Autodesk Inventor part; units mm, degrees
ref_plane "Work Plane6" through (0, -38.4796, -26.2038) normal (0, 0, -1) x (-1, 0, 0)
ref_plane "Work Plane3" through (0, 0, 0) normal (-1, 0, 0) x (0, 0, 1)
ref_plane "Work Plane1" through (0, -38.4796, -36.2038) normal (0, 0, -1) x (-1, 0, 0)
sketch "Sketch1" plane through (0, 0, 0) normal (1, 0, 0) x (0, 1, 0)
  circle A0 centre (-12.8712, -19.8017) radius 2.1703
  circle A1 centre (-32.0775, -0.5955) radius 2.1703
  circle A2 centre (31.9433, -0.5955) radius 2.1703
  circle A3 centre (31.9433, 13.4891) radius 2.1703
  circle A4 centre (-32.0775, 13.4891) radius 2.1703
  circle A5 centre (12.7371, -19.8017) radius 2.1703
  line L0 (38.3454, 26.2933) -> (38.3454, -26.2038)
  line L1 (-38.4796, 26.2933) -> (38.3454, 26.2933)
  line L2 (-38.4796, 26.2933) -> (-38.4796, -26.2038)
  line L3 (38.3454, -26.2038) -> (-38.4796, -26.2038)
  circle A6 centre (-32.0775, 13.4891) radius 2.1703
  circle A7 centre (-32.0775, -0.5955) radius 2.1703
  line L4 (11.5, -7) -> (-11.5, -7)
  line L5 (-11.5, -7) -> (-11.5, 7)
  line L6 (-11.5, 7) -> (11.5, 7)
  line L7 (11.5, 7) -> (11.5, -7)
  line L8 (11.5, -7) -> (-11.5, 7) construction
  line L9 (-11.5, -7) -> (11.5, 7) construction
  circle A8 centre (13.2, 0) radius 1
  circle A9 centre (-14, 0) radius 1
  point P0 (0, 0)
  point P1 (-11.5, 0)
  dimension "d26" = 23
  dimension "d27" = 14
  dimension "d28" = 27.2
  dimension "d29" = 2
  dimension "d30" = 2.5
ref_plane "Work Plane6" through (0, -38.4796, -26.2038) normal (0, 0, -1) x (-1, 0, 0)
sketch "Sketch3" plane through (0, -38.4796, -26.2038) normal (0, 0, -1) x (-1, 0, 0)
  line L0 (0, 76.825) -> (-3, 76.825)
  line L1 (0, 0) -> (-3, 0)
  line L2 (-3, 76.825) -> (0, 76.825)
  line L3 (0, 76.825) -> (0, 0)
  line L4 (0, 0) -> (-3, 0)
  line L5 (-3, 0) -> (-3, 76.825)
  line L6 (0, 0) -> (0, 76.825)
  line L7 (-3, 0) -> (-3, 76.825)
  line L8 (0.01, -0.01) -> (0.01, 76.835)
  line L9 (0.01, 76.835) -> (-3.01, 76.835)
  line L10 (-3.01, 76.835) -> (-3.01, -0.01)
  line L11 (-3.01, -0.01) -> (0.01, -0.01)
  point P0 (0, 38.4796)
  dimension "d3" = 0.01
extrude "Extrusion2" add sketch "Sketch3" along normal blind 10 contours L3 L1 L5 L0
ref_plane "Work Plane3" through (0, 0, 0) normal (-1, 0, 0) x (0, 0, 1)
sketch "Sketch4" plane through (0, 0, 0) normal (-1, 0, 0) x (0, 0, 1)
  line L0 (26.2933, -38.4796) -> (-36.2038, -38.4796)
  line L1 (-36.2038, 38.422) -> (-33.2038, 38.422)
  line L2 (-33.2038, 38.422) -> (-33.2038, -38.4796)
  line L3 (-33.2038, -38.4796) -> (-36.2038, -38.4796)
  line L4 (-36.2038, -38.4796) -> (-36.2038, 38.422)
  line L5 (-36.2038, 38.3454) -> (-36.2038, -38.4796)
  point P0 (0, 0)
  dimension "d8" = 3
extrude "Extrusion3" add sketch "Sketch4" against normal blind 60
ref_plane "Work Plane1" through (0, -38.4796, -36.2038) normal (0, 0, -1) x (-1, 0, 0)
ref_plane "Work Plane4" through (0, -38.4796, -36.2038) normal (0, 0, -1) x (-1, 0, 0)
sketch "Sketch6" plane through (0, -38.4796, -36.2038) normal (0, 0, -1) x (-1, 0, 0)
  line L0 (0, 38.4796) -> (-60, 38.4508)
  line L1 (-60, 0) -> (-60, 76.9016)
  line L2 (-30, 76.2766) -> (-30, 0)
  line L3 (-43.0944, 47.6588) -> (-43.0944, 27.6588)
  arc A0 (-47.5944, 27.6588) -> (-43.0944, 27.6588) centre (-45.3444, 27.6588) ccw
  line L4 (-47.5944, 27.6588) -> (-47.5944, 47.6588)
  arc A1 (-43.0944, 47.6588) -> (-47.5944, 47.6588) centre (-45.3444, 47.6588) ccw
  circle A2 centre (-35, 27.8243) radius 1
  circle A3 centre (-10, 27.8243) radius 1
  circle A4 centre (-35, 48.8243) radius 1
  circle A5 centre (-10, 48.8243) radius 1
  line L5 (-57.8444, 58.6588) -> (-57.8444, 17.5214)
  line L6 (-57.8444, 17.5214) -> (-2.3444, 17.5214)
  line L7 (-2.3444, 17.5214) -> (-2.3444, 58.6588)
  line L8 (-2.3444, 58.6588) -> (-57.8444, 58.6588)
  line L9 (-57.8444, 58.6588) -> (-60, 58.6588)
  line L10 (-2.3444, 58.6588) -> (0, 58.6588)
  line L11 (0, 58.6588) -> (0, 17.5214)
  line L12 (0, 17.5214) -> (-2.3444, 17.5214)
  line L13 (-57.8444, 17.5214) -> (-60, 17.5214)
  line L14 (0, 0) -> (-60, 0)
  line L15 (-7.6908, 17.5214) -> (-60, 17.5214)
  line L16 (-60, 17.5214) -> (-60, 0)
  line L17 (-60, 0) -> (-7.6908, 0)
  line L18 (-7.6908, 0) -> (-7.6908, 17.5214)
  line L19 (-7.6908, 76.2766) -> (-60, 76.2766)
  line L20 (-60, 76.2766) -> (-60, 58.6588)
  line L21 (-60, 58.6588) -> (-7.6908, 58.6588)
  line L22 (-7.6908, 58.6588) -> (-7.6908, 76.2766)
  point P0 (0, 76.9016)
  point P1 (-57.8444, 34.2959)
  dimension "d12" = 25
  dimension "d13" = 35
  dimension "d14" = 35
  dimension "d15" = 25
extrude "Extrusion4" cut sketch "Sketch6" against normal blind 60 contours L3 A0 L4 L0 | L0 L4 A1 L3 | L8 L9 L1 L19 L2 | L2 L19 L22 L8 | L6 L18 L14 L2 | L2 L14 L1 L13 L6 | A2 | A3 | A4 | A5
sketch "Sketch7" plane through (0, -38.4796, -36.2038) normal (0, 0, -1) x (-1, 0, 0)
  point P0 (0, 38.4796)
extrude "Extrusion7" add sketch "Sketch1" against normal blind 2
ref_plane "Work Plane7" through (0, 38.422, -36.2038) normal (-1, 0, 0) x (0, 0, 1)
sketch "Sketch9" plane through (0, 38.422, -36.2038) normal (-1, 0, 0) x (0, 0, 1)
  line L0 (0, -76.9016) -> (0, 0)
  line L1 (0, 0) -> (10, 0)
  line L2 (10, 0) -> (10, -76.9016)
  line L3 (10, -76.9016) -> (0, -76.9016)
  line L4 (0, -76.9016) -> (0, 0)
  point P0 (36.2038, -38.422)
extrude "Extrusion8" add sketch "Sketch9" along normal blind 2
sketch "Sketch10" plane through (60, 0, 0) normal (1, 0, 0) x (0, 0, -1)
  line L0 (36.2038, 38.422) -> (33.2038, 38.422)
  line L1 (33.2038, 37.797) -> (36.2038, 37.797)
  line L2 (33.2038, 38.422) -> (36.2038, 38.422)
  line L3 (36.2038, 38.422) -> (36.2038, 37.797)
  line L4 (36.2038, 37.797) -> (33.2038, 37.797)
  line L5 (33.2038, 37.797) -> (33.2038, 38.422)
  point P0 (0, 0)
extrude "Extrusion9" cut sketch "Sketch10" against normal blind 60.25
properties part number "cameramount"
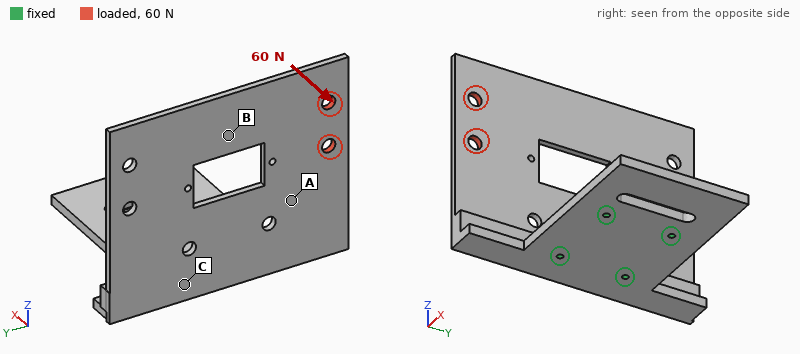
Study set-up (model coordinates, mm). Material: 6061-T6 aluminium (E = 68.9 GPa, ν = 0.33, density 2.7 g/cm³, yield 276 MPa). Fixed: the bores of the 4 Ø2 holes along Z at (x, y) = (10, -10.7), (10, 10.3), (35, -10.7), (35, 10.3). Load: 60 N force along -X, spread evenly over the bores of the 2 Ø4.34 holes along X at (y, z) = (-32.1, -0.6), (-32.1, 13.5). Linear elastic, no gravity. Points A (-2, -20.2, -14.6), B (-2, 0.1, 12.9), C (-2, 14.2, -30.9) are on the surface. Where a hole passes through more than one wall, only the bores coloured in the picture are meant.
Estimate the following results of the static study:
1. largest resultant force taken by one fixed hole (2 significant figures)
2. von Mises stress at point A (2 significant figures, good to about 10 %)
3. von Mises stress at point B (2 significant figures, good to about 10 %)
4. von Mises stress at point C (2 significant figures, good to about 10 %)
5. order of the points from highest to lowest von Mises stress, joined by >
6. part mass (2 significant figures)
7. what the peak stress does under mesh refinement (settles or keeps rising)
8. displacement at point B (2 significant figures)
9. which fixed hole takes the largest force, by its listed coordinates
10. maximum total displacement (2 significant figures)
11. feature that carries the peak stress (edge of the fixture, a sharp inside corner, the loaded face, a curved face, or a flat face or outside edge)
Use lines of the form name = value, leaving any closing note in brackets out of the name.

largest resultant force taken by one fixed hole = 72 N
von Mises stress at point A = 42 MPa
von Mises stress at point B = 17 MPa
von Mises stress at point C = 8.4 MPa
order of the points from highest to lowest von Mises stress, joined by > = A > B > C
part mass = 49 g
what the peak stress does under mesh refinement = keeps rising
displacement at point B = 0.46 mm
which fixed hole takes the largest force, by its listed coordinates = (10, -10.7)
maximum total displacement = 1.1 mm
feature that carries the peak stress = edge of the fixture
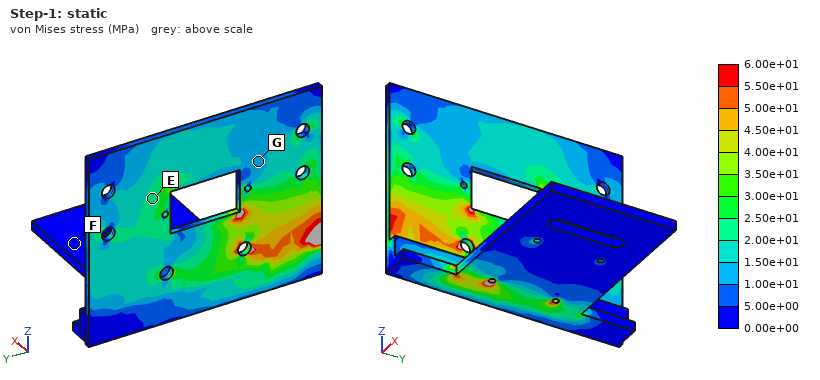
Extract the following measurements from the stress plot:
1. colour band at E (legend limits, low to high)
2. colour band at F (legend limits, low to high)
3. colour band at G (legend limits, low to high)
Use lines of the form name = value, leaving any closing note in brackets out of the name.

colour band at E = 2.00e+01 to 2.50e+01 MPa
colour band at F = 0.00e+00 to 5.00e+00 MPa
colour band at G = 1.00e+01 to 1.50e+01 MPa
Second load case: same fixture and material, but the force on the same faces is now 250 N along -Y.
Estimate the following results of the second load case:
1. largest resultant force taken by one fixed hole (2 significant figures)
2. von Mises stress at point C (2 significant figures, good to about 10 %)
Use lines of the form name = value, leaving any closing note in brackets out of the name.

largest resultant force taken by one fixed hole = 470 N
von Mises stress at point C = 19 MPa
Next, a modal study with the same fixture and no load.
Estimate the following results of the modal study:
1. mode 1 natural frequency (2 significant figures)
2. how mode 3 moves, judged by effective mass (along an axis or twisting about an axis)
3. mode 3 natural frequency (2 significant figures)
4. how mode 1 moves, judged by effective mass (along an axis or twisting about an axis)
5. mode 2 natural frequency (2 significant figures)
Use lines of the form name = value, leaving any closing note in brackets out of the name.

mode 1 natural frequency = 450 Hz
how mode 3 moves, judged by effective mass = along Y
mode 3 natural frequency = 1600 Hz
how mode 1 moves, judged by effective mass = along X
mode 2 natural frequency = 920 Hz
